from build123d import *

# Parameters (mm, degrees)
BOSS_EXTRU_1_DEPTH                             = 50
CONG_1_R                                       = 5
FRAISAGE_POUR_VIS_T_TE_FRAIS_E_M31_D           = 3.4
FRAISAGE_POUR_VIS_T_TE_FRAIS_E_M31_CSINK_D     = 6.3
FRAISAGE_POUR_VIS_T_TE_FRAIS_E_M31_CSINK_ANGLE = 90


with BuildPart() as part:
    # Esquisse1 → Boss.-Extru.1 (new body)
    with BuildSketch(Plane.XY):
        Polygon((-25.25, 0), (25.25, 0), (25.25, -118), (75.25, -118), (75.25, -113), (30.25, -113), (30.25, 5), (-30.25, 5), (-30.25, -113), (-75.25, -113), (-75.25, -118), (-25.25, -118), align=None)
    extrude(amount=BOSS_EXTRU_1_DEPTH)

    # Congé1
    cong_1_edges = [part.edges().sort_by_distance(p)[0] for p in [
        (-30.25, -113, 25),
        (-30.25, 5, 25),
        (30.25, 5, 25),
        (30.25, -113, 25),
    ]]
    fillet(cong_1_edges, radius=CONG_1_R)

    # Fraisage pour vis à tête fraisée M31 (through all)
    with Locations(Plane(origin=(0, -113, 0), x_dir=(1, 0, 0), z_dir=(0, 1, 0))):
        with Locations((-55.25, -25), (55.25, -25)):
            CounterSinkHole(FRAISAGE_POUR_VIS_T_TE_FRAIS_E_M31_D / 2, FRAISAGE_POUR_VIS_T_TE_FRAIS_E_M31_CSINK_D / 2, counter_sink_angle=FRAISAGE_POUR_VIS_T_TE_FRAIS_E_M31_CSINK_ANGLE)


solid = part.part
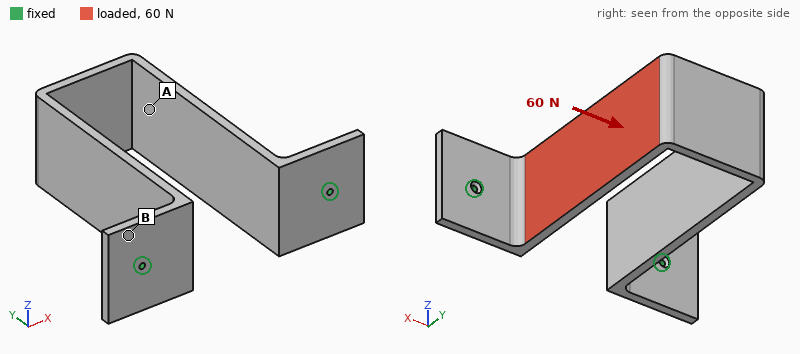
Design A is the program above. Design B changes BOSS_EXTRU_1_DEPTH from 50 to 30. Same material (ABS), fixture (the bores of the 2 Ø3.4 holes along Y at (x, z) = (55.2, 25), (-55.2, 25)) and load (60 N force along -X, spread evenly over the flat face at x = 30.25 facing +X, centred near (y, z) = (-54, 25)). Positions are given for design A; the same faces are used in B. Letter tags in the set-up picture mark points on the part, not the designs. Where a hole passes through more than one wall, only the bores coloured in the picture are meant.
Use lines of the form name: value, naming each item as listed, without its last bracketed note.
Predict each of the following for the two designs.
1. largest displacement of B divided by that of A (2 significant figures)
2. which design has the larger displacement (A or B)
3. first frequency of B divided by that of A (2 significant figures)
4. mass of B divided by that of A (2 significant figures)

largest displacement of B divided by that of A: 1.7
which design has the larger displacement: B
first frequency of B divided by that of A: 0.99
mass of B divided by that of A: 0.60
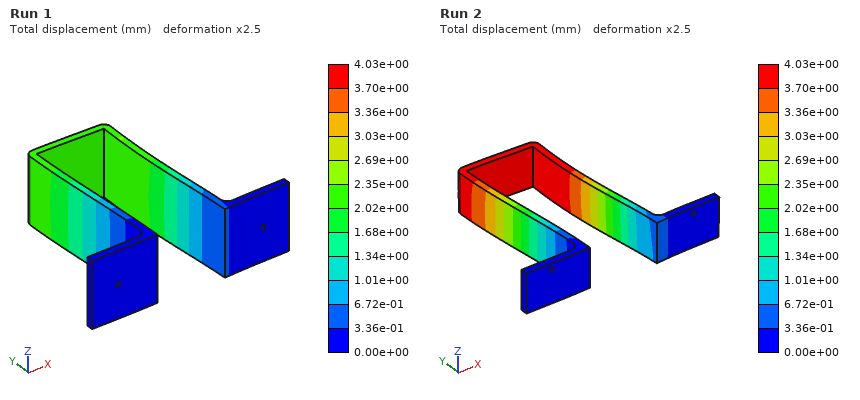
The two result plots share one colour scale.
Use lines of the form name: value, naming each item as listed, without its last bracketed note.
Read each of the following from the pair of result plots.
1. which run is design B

which run is design B: Run 2
